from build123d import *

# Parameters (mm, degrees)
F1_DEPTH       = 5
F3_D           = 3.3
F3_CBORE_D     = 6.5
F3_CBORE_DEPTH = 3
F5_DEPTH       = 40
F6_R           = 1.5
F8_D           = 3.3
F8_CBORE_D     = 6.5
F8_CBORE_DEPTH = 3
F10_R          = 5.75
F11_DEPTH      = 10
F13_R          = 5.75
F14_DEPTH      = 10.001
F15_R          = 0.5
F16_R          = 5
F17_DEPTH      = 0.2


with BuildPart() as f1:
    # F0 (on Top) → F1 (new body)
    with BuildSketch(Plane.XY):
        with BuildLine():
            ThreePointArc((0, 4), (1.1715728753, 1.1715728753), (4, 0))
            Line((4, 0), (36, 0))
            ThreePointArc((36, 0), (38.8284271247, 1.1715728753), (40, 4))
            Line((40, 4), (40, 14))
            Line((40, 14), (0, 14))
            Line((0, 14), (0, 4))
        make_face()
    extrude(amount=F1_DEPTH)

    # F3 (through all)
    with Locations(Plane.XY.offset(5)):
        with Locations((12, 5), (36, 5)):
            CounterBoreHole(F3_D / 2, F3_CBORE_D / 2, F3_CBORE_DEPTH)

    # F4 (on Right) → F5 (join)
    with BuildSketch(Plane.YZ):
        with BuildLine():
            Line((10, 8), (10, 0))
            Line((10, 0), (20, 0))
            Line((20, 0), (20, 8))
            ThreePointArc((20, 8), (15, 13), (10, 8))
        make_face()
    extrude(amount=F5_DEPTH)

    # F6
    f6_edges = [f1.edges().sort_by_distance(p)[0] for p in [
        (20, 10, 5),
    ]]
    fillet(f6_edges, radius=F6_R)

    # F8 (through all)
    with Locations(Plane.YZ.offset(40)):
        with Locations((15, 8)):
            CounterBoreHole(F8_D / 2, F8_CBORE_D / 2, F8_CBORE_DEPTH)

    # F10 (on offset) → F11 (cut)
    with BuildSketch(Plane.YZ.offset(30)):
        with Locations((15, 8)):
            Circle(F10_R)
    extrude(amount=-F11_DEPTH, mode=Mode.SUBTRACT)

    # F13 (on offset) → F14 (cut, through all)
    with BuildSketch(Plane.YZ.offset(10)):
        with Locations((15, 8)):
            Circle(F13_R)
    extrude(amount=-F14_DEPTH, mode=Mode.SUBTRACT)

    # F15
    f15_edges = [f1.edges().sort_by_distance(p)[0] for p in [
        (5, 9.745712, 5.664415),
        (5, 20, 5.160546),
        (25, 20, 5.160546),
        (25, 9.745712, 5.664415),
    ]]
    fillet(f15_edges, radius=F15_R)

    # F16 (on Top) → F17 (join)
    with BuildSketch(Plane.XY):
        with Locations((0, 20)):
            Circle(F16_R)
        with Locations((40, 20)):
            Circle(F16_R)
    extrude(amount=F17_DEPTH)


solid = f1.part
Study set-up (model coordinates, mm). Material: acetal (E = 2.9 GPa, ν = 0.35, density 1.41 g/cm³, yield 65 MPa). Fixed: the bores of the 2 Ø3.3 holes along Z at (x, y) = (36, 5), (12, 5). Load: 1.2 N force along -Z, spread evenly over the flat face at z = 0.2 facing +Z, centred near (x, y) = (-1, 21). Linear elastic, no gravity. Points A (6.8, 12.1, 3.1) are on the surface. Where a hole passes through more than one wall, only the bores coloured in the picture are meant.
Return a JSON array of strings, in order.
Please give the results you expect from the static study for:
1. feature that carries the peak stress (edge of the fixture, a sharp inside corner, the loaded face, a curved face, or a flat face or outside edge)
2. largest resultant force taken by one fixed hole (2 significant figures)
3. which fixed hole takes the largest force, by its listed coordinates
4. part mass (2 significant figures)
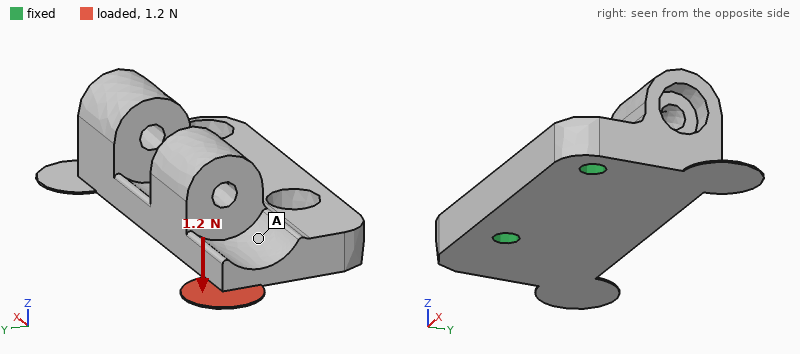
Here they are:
["a flat face or outside edge", "1.8 N", "(12, 5)", "6.4 g"]
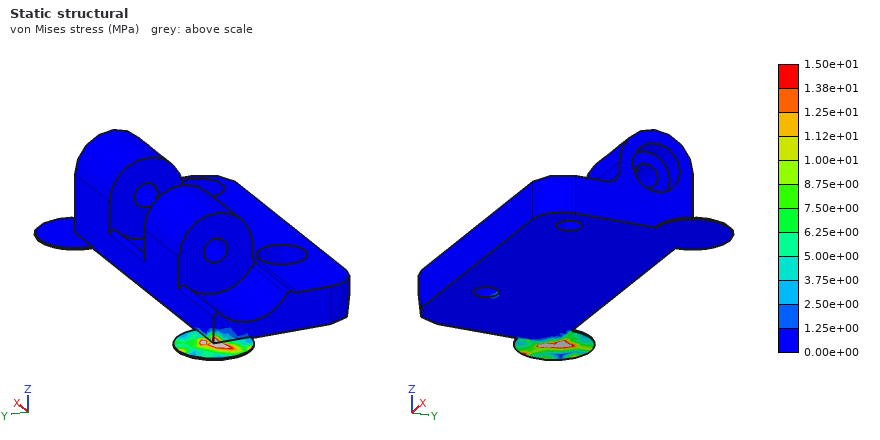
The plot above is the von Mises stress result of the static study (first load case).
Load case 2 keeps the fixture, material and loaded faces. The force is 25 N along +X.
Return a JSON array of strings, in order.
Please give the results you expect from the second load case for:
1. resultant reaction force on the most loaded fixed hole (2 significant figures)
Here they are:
["20 N"]
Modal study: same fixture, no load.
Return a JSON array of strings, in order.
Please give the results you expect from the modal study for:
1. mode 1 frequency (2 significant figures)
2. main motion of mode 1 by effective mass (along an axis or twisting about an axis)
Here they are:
["1600 Hz", "along Z"]
